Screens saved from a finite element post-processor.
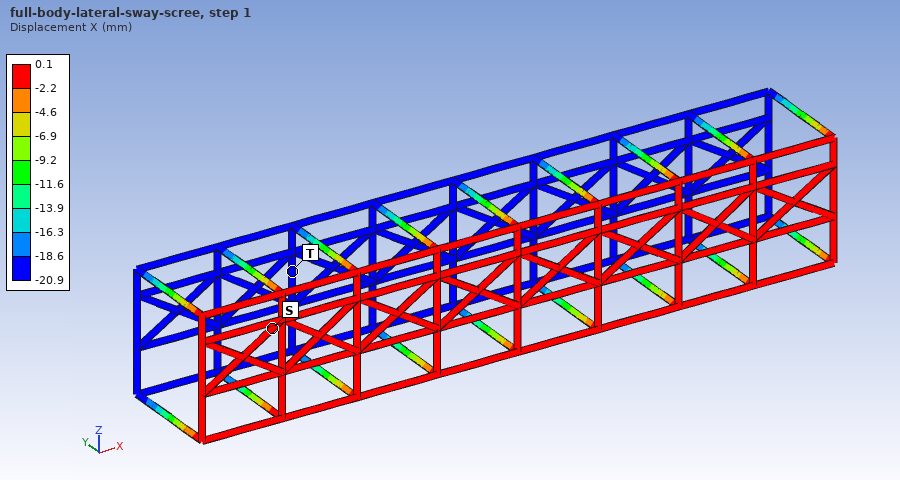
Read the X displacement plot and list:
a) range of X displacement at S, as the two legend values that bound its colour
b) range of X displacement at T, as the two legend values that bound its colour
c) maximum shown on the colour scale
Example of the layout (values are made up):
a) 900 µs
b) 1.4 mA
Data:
a) -2.2 to 0.1 mm
b) -20.9 to -18.6 mm
c) 0.1 mm
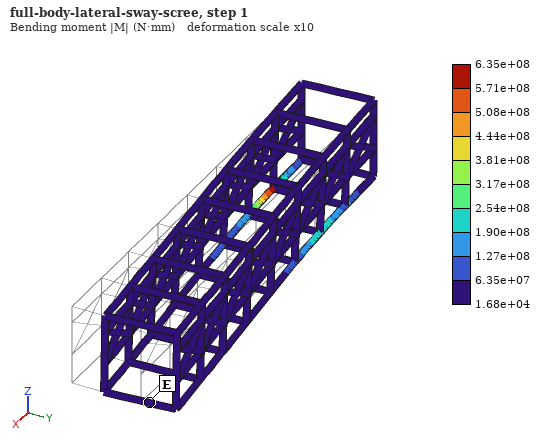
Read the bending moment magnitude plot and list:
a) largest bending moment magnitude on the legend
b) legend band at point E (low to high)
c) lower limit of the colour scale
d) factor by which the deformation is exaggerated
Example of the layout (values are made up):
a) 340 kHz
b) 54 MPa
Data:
a) 6.35e+08 N·mm
b) 1.68e+04 to 6.35e+07 N·mm
c) 1.68e+04 N·mm
d) 10
